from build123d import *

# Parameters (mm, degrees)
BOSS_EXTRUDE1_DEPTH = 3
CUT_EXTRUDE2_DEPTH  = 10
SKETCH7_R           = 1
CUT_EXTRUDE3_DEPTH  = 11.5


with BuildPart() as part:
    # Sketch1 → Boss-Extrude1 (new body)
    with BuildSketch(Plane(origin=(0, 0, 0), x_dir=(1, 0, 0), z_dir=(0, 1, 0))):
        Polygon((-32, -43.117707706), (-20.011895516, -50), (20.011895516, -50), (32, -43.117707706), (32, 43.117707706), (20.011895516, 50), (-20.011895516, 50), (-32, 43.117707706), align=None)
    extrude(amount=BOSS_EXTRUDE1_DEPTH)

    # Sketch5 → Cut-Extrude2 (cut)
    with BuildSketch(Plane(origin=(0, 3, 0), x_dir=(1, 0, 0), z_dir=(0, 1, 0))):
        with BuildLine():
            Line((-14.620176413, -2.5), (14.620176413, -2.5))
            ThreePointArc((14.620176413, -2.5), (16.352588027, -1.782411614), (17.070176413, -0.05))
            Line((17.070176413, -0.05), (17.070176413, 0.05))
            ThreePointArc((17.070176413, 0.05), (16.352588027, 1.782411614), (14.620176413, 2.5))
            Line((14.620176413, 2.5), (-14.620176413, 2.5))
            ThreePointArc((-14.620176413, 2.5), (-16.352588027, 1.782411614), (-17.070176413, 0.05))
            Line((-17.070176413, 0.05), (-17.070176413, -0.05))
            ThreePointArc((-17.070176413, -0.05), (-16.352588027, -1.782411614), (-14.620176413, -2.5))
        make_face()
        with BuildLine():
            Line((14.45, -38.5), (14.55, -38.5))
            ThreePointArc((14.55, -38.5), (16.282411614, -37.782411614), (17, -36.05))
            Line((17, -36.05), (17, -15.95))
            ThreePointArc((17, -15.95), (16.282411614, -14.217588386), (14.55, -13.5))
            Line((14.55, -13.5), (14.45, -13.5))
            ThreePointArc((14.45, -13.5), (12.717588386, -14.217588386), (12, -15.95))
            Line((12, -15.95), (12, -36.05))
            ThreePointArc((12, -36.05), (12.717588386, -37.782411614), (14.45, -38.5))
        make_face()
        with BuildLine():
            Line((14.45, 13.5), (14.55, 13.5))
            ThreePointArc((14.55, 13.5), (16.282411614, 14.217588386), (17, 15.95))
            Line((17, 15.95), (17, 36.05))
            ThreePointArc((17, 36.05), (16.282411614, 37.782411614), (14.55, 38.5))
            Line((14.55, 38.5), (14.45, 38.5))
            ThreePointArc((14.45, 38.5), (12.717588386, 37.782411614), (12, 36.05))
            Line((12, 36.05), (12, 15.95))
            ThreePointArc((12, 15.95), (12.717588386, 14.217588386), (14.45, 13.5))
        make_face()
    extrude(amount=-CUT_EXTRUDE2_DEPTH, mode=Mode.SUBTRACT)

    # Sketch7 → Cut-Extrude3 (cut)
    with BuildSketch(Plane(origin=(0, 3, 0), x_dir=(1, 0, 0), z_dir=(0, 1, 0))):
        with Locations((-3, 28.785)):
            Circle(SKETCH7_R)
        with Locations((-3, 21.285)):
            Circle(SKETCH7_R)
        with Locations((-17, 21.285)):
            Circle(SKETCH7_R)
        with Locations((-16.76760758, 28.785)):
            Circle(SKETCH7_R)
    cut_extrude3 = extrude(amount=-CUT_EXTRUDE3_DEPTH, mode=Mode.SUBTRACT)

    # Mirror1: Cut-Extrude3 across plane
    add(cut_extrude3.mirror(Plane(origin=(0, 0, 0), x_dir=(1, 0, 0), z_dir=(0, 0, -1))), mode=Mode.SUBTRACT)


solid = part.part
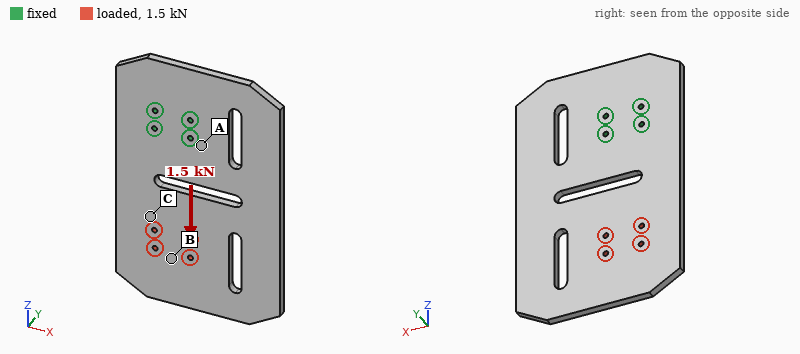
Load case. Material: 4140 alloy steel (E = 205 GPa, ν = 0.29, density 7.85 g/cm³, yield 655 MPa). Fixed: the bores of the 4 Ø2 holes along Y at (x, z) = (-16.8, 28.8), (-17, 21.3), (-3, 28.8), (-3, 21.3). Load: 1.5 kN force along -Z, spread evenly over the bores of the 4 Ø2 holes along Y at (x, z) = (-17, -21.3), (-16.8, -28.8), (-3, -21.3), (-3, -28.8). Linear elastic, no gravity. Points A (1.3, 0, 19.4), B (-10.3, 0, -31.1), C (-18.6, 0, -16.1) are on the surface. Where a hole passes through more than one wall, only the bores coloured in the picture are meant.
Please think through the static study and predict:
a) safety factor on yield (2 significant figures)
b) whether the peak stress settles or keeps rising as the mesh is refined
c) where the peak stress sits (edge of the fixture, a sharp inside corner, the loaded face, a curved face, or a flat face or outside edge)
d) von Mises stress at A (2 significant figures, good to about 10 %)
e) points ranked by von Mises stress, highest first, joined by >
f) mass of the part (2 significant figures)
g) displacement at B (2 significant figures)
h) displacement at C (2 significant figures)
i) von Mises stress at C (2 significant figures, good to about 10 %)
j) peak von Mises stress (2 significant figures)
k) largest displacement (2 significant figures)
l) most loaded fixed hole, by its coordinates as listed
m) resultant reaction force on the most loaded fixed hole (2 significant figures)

6.4
settles
a curved face
9.4 MPa
C > A > B
140 g
6.4 µm
4.9 µm
21 MPa
100 MPa
7.0 µm
(-17, 21.3)
540 N
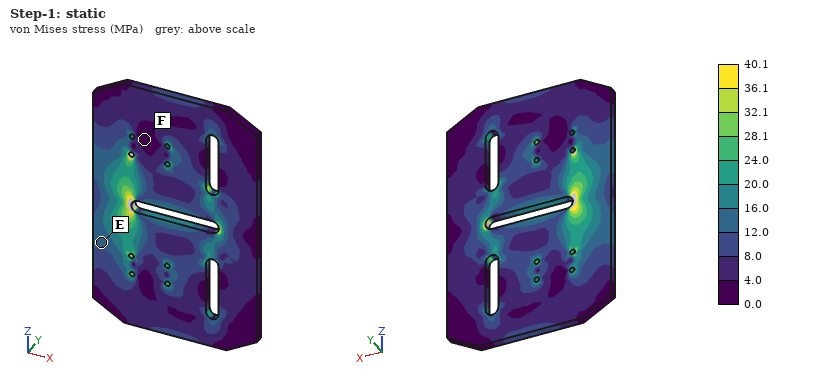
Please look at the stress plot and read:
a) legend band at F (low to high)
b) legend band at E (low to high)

0.0 to 4.0 MPa
12.0 to 16.0 MPa
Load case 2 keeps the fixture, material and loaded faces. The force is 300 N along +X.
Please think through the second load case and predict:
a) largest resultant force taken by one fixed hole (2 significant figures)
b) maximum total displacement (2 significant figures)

540 N
12 µm
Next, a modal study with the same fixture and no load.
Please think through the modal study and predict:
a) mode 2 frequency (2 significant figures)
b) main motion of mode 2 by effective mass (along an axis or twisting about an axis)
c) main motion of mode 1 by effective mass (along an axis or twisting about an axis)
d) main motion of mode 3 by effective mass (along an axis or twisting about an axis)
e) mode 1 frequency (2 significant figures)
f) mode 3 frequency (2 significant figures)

1000 Hz
twisting about Z
along Y
along Y
390 Hz
1900 Hz
